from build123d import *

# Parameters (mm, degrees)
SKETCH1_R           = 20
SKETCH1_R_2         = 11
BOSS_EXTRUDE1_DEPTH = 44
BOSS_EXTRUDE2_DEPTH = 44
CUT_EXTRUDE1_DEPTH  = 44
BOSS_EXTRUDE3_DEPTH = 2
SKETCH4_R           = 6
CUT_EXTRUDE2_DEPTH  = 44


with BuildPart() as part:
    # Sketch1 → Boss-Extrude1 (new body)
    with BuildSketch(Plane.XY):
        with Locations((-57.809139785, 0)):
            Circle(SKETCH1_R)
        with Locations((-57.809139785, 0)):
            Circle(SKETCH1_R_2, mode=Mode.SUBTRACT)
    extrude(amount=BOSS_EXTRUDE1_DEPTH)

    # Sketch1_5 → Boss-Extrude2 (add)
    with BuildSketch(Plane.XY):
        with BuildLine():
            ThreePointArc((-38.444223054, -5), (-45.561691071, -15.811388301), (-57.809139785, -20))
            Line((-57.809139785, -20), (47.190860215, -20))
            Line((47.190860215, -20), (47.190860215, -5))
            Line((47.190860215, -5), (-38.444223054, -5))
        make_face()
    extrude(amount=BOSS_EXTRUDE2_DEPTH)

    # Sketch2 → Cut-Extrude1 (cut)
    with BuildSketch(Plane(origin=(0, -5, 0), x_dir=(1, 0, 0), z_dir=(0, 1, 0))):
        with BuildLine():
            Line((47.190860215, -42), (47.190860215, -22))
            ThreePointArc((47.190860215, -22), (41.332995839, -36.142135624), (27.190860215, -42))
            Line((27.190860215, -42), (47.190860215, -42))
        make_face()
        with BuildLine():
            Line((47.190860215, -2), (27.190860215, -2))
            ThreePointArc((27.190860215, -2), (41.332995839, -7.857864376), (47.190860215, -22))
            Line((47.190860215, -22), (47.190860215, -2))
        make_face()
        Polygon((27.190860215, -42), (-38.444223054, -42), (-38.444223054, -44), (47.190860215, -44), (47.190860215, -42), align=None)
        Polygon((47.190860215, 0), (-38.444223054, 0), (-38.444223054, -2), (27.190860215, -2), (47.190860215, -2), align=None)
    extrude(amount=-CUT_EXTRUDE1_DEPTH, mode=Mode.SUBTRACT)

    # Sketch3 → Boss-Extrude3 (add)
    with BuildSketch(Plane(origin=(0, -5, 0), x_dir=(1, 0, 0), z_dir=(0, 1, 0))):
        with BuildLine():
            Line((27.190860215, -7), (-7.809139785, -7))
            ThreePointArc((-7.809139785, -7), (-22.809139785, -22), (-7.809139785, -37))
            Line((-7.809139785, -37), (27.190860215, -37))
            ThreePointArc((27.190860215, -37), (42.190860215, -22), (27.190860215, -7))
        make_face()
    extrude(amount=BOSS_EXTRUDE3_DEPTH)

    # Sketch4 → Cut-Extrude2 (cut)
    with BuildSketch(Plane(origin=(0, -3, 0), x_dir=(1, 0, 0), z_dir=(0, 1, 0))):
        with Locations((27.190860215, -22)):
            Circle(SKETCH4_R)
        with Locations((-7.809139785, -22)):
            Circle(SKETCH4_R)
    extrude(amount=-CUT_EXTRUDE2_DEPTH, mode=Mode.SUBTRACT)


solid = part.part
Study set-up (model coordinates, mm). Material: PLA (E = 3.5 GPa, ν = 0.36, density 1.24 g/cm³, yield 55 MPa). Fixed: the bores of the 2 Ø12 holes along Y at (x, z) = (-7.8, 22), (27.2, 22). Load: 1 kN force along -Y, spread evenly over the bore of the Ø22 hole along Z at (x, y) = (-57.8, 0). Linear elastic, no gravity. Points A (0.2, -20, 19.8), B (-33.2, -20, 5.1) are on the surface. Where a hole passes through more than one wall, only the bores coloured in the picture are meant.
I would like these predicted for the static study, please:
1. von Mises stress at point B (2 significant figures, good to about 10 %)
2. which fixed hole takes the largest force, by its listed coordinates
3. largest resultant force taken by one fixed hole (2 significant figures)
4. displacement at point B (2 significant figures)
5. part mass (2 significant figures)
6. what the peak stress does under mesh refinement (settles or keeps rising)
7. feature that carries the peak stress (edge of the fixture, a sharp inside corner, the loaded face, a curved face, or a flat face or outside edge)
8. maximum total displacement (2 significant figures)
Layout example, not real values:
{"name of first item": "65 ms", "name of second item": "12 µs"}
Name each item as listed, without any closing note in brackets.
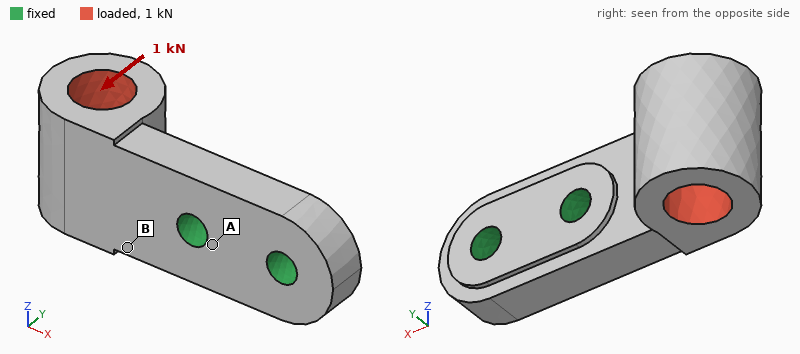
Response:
{"von Mises stress at point B": "16 MPa", "which fixed hole takes the largest force, by its listed coordinates": "(-7.8, 22)", "largest resultant force taken by one fixed hole": "1.2 kN", "displacement at point B": "0.30 mm", "part mass": "110 g", "what the peak stress does under mesh refinement": "keeps rising", "feature that carries the peak stress": "edge of the fixture", "maximum total displacement": "1.5 mm"}
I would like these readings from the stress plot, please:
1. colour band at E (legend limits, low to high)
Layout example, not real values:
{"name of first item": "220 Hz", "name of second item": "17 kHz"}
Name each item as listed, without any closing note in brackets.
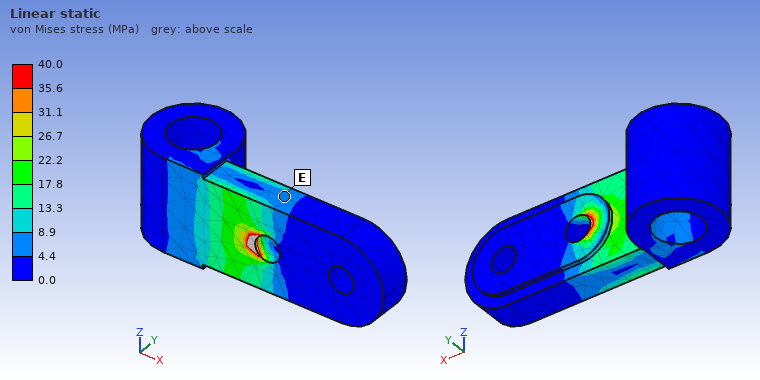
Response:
{"colour band at E": "4.4 to 8.9 MPa"}
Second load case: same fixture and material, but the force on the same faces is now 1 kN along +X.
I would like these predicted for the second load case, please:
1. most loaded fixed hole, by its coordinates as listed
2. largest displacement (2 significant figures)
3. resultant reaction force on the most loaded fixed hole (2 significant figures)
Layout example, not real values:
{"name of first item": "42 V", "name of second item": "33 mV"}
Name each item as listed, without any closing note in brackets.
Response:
{"most loaded fixed hole, by its coordinates as listed": "(-7.8, 22)", "largest displacement": "0.59 mm", "resultant reaction force on the most loaded fixed hole": "890 N"}
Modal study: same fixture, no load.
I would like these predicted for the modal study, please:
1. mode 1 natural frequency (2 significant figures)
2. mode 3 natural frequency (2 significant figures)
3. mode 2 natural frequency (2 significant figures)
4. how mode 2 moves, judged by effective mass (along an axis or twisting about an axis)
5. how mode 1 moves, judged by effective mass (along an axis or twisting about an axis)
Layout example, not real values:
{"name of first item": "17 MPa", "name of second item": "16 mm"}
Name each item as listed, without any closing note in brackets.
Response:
{"mode 1 natural frequency": "650 Hz", "mode 3 natural frequency": "1800 Hz", "mode 2 natural frequency": "1000 Hz", "how mode 2 moves, judged by effective mass": "along Z", "how mode 1 moves, judged by effective mass": "along Y"}
